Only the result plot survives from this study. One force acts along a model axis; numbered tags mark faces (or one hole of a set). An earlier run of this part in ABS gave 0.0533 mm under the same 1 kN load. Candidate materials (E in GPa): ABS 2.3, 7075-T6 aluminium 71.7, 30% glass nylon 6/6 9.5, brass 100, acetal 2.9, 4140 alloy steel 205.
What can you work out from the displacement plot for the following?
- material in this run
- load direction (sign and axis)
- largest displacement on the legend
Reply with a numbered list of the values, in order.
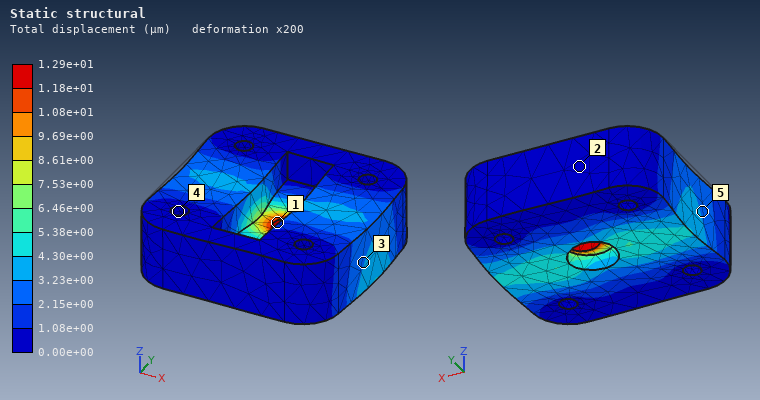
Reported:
1. 30% glass nylon 6/6
2. +X
3. 1.29e+01 µm
